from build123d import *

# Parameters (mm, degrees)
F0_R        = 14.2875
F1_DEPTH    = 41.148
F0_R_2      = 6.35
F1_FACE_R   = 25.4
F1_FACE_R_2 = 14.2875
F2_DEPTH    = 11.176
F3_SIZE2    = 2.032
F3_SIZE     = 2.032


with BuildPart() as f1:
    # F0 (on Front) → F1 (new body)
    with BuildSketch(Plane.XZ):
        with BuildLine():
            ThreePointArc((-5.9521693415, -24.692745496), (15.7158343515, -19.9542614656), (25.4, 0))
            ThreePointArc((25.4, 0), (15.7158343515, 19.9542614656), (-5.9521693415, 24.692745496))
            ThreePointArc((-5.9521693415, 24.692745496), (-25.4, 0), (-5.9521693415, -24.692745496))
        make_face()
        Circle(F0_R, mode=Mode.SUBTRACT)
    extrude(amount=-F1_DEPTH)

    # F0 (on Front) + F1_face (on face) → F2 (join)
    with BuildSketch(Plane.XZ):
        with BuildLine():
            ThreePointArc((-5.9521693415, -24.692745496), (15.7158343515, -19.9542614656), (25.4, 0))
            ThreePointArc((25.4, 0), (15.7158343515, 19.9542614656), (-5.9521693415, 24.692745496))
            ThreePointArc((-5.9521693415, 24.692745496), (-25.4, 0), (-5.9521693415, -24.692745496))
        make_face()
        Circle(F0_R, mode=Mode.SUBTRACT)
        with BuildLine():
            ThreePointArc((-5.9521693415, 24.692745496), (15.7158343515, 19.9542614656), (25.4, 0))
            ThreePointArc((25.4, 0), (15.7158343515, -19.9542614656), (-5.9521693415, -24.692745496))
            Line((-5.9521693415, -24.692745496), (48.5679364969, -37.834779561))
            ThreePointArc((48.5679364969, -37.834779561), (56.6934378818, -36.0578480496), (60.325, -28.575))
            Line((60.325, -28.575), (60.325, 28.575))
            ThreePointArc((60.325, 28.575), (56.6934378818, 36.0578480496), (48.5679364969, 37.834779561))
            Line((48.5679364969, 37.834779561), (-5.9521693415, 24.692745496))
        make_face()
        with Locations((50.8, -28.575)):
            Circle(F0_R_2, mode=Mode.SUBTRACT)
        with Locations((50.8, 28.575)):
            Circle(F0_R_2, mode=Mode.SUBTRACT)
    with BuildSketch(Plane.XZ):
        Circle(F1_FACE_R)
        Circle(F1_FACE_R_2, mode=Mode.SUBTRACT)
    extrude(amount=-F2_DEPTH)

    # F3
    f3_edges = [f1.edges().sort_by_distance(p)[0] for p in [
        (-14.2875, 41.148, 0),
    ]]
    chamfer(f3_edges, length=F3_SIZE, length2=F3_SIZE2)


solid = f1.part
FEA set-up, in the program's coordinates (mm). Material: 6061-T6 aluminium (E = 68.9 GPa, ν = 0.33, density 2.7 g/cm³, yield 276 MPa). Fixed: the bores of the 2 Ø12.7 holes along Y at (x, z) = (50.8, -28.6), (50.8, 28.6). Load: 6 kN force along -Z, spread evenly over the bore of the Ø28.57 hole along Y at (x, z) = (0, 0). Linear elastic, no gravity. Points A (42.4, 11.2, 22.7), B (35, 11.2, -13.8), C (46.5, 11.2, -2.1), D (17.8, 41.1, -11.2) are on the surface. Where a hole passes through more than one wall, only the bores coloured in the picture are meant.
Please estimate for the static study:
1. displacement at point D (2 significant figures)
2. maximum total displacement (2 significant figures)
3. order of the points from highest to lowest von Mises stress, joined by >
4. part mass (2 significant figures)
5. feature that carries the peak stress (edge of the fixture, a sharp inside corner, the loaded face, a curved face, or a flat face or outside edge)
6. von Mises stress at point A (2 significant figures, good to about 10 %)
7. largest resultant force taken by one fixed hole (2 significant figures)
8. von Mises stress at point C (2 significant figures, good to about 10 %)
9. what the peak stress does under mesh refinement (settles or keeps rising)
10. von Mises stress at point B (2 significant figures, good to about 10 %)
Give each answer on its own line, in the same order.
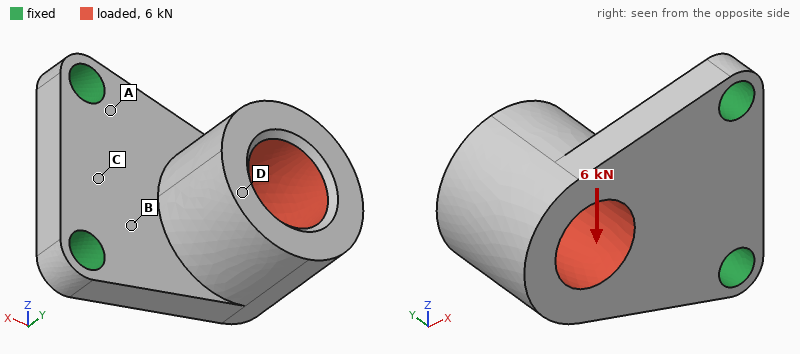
70 µm
94 µm
B > A > C > D
230 g
edge of the fixture
24 MPa
6.0 kN
15 MPa
keeps rising
34 MPa
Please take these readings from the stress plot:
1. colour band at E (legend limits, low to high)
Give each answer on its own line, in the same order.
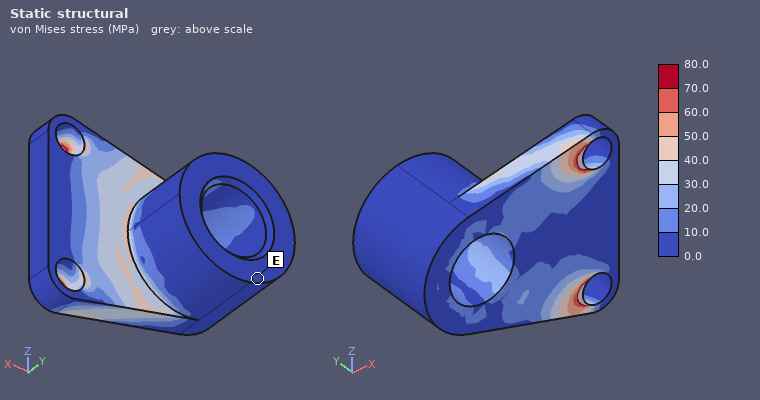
0.0 to 10.0 MPa
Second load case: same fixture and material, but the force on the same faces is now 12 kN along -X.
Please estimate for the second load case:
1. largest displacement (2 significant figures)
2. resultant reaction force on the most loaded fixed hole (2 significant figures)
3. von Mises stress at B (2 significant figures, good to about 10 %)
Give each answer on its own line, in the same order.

0.72 mm
6.4 kN
110 MPa
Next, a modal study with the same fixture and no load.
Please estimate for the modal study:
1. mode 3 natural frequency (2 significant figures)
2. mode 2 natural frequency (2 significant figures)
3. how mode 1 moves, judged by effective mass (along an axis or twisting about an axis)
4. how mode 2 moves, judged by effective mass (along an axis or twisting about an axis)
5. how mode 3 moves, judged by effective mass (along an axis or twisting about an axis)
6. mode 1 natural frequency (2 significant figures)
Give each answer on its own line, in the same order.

6100 Hz
3500 Hz
along Y
along Z
along Z
1200 Hz
